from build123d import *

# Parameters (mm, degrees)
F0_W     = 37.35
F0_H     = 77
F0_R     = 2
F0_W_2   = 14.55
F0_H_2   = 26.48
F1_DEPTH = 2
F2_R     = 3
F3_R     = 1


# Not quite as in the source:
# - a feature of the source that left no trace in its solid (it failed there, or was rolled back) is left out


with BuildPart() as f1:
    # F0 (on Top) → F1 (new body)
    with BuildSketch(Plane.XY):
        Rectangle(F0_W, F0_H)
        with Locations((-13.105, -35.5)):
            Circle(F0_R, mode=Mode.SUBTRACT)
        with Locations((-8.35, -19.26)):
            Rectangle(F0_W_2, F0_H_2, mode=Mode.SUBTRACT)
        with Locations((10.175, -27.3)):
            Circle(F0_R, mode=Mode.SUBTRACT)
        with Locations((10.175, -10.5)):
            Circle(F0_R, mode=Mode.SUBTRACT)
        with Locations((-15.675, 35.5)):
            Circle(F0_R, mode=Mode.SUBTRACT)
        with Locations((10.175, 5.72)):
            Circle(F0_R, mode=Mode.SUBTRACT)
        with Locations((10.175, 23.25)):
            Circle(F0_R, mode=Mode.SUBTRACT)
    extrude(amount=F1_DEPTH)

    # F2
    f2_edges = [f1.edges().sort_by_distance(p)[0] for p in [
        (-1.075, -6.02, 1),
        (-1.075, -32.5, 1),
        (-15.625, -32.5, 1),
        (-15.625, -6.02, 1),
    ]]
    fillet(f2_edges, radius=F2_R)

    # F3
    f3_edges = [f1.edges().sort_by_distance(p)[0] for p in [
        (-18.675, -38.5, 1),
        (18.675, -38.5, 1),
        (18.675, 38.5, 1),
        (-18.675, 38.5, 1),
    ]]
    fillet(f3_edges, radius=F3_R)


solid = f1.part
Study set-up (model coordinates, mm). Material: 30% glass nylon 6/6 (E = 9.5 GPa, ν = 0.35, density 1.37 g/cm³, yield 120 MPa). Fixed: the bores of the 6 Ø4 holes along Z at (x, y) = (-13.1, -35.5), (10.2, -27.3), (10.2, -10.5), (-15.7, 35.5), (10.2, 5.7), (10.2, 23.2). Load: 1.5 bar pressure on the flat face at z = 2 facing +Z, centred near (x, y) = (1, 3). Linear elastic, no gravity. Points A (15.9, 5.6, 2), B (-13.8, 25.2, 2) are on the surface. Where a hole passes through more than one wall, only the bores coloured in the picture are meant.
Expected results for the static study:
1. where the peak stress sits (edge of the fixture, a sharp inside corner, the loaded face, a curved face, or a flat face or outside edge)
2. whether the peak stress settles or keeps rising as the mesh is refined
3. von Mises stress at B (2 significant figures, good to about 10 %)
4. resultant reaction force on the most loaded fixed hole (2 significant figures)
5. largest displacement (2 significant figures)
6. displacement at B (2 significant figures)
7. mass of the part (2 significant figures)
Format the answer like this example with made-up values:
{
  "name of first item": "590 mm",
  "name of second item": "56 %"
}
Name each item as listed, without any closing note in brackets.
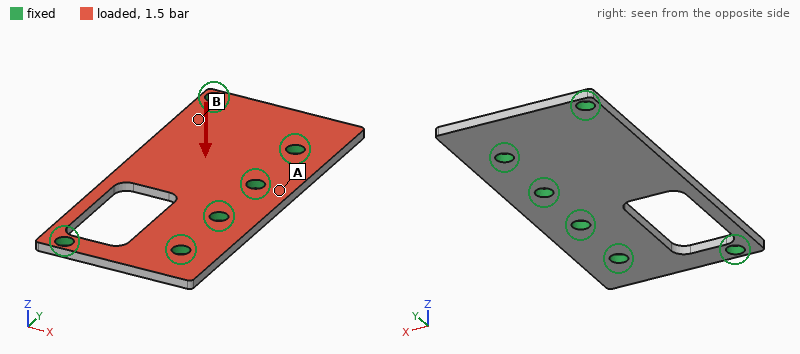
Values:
{
  "where the peak stress sits": "edge of the fixture",
  "whether the peak stress settles or keeps rising as the mesh is refined": "keeps rising",
  "von Mises stress at B": "20 MPa",
  "resultant reaction force on the most loaded fixed hole": "82 N",
  "largest displacement": "0.78 mm",
  "displacement at B": "0.15 mm",
  "mass of the part": "6.6 g"
}
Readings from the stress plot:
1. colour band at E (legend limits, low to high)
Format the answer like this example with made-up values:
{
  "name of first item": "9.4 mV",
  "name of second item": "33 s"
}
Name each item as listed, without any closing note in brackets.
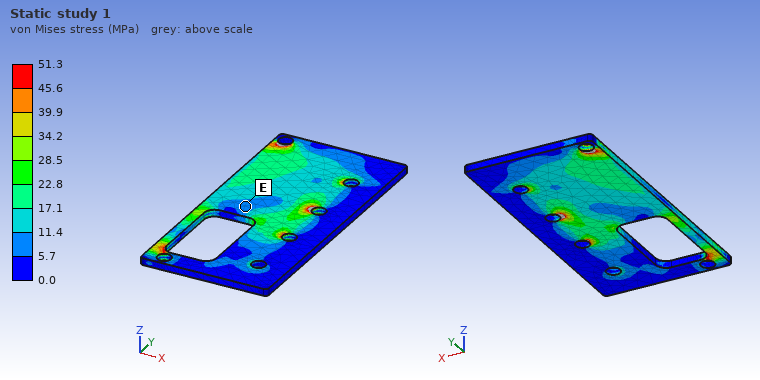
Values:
{
  "colour band at E": "5.7 to 11.4 MPa"
}
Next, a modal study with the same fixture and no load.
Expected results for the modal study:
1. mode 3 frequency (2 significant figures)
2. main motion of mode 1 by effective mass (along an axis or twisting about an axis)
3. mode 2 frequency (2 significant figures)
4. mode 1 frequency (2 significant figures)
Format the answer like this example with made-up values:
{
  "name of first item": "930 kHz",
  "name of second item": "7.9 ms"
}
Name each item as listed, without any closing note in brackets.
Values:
{
  "mode 3 frequency": "4600 Hz",
  "main motion of mode 1 by effective mass": "along Z",
  "mode 2 frequency": "3800 Hz",
  "mode 1 frequency": "1800 Hz"
}
